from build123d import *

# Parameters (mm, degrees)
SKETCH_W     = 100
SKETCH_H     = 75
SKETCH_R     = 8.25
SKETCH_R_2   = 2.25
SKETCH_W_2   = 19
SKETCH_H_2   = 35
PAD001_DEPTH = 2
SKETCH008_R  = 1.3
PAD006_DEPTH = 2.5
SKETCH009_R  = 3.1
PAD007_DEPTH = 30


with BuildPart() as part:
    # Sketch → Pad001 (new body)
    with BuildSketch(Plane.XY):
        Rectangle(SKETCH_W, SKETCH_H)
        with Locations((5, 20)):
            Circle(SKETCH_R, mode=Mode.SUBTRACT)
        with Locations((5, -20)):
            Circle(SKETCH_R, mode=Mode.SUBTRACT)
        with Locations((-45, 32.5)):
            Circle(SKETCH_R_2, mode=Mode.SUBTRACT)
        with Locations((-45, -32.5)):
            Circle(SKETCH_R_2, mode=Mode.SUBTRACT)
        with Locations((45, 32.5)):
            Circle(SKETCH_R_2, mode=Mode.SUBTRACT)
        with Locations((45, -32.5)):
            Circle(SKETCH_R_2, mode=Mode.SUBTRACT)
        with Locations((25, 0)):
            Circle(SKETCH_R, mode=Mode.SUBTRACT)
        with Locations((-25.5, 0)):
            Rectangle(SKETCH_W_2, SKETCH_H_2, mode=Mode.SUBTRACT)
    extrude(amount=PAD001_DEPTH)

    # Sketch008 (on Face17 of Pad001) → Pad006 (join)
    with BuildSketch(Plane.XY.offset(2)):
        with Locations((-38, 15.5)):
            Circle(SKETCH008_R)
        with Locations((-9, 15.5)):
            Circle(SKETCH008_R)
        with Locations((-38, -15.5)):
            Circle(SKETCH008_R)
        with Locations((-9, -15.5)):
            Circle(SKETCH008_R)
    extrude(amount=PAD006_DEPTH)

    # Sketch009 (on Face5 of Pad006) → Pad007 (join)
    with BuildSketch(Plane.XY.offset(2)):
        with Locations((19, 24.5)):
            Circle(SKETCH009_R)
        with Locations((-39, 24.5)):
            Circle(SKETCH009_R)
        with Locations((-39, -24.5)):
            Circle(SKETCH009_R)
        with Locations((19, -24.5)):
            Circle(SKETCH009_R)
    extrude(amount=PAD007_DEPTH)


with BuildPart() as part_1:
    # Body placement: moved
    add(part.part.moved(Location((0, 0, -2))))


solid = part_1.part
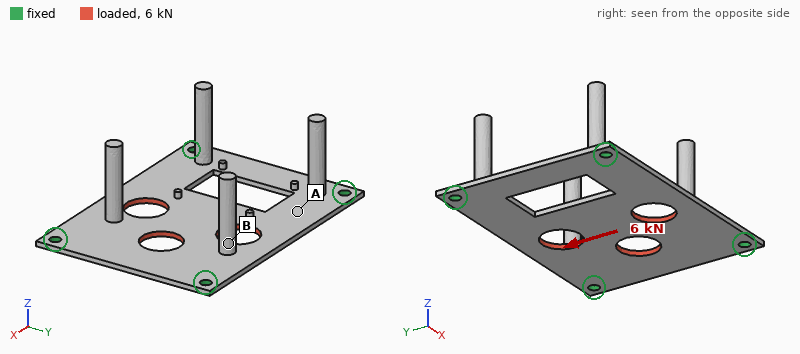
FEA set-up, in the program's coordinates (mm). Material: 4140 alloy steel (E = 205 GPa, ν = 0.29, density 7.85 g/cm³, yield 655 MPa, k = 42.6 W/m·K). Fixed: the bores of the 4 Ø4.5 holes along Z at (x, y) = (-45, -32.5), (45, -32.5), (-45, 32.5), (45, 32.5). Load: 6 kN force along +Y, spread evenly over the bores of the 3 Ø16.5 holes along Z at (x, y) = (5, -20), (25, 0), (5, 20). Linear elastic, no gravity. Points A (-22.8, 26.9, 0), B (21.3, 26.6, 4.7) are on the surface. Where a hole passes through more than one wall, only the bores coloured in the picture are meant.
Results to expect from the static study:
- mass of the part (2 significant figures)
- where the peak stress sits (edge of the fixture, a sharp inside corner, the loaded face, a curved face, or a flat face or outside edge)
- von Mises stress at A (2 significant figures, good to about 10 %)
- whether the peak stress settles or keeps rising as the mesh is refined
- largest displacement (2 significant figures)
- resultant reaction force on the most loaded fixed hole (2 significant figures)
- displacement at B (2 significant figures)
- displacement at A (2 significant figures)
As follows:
130 g
edge of the fixture
46 MPa
keeps rising
27 µm
2.7 kN
18 µm
15 µm
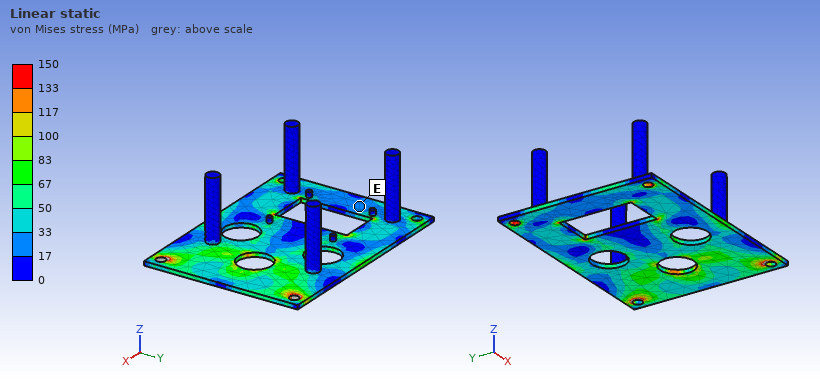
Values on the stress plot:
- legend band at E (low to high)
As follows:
17 to 33 MPa
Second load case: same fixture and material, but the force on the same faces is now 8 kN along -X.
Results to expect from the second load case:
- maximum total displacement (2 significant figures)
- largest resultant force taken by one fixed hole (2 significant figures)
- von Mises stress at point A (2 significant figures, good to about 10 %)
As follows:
17 µm
2.6 kN
43 MPa
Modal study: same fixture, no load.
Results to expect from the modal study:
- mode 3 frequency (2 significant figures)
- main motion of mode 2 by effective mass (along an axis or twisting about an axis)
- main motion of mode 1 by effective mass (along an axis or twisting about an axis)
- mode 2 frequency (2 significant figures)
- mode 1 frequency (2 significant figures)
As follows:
1600 Hz
twisting about X
along Z
1300 Hz
900 Hz
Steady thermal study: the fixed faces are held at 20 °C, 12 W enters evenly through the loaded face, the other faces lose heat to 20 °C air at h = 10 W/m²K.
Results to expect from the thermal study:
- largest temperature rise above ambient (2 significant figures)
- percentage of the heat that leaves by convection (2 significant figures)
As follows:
49 K
30 %
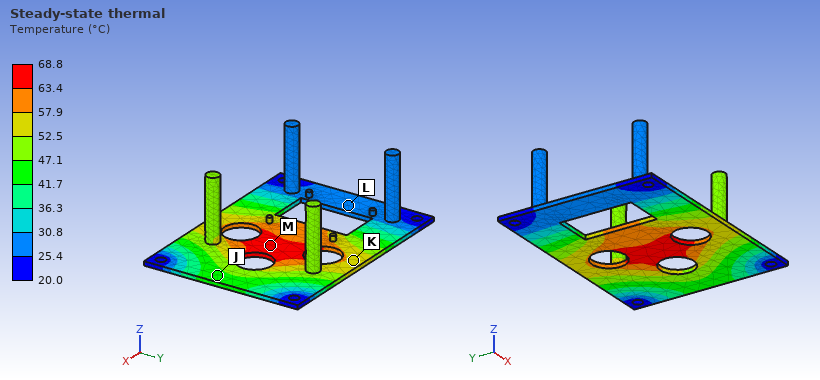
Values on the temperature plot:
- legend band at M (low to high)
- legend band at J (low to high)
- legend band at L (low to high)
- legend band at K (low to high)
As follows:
63.4 to 68.8 °C
41.7 to 47.1 °C
25.4 to 30.8 °C
52.5 to 57.9 °C
